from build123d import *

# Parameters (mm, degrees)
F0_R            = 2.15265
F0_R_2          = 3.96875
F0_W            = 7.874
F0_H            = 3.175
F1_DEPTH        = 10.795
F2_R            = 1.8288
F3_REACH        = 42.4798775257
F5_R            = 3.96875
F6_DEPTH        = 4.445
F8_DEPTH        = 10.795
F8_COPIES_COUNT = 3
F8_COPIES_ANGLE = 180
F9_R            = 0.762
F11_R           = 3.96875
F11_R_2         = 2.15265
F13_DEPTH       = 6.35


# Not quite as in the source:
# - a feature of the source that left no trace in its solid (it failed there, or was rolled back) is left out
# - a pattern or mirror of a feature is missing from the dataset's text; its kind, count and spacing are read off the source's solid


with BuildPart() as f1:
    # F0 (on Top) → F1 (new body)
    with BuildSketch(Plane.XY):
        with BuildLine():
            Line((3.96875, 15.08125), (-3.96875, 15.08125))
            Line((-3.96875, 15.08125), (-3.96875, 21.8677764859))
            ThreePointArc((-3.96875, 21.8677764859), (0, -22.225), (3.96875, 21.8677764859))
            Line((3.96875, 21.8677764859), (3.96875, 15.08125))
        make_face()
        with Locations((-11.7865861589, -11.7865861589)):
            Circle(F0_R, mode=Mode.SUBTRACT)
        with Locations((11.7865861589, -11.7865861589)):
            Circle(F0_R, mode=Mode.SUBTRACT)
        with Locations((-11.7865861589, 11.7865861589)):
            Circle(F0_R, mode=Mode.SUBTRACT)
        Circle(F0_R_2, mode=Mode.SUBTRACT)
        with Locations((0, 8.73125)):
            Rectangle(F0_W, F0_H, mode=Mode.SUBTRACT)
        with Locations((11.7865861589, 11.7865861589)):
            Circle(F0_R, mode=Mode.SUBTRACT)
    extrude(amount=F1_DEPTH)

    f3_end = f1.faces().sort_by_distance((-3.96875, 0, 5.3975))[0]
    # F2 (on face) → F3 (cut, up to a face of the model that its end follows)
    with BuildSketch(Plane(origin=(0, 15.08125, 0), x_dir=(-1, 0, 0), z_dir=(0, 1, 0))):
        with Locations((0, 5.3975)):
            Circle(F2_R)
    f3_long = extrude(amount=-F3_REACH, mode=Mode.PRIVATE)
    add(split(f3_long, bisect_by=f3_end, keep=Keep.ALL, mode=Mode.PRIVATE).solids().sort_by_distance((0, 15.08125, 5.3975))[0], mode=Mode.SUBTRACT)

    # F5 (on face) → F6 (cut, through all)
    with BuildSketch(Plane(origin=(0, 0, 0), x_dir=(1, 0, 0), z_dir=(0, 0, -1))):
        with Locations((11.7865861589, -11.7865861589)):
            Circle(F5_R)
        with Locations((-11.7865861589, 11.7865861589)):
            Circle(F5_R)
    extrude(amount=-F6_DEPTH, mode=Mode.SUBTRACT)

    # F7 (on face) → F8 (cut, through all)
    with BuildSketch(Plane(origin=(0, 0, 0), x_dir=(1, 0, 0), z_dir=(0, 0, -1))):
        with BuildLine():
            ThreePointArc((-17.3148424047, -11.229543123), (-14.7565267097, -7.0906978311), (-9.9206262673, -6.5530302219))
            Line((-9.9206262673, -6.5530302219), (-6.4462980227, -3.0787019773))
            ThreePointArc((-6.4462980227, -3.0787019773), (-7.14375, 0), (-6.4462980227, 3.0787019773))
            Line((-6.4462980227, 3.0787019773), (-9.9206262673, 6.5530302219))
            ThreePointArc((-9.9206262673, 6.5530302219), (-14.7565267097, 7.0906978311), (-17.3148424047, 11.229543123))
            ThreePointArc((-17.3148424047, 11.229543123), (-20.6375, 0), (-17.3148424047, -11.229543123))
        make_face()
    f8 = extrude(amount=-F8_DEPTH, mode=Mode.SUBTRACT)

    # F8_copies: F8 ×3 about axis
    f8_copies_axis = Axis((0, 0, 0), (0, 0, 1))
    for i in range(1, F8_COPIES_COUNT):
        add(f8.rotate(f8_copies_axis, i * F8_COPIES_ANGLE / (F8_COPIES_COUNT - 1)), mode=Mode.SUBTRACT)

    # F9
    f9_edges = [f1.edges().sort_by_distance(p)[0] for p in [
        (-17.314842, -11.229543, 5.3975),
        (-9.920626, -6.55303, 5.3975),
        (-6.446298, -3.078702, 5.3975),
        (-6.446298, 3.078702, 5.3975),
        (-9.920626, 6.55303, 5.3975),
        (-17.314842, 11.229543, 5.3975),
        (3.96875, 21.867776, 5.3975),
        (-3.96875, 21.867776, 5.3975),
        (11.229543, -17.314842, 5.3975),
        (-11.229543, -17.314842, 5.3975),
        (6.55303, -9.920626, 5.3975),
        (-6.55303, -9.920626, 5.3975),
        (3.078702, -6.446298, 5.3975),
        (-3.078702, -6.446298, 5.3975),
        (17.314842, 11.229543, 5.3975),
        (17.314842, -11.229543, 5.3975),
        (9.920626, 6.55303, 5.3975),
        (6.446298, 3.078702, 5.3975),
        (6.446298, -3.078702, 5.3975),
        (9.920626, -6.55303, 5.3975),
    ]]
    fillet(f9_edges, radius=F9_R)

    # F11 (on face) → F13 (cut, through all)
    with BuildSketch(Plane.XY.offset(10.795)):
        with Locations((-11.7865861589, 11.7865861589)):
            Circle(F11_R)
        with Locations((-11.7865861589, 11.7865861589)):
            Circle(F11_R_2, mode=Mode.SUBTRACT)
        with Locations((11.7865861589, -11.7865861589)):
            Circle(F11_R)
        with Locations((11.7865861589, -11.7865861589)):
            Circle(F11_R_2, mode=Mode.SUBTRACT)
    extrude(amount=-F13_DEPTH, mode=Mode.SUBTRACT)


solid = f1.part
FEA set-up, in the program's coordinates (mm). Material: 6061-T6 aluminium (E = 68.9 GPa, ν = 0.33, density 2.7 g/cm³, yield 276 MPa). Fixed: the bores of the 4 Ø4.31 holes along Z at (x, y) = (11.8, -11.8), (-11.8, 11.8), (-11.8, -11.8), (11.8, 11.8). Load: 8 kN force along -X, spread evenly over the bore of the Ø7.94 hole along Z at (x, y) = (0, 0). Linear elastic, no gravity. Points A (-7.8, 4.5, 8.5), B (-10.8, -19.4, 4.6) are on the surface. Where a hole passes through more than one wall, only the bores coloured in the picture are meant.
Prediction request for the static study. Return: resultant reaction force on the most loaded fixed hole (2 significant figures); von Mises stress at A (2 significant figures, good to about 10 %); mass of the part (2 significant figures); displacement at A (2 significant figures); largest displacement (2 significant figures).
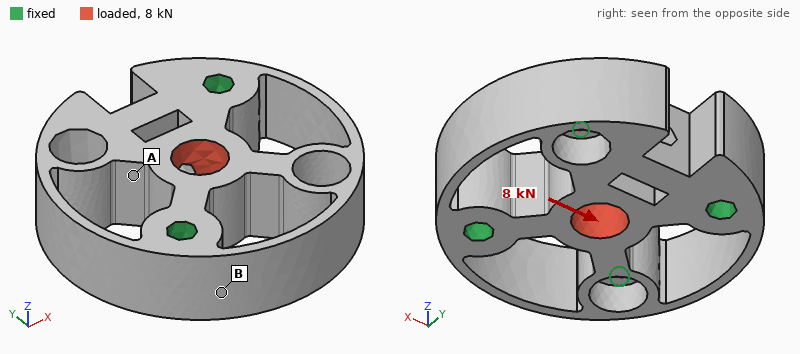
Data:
2.5 kN
40 MPa
21 g
13 µm
20 µm
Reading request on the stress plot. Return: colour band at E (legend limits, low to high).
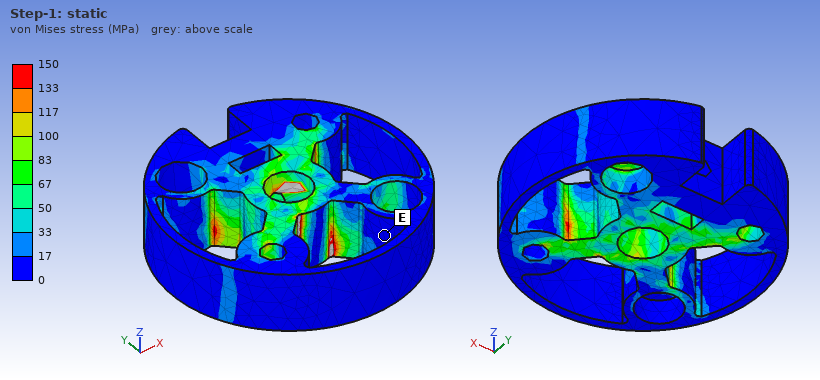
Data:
0 to 17 MPa
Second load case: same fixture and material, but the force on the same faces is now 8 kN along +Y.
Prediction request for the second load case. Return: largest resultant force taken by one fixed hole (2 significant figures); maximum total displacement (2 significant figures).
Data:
2.5 kN
20 µm
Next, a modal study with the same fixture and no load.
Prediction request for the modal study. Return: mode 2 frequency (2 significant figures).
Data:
26 kHz
